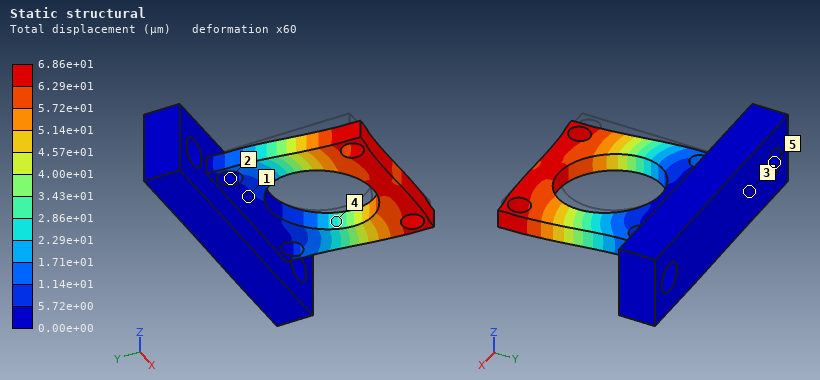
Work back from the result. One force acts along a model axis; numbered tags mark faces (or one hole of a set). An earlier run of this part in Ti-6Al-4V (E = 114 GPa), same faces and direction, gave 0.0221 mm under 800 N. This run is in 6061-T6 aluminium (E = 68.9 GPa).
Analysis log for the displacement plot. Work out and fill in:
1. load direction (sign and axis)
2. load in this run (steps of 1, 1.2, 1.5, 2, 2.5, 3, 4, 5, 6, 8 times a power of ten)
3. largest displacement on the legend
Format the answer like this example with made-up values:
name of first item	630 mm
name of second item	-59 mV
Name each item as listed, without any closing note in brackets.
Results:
load direction	+X
load in this run	1.5 kN
largest displacement on the legend	6.86e+01 µm
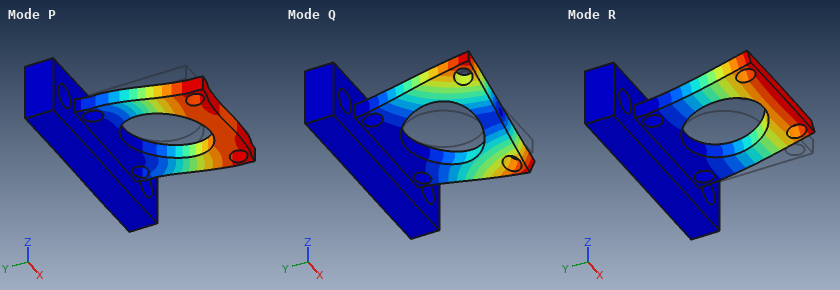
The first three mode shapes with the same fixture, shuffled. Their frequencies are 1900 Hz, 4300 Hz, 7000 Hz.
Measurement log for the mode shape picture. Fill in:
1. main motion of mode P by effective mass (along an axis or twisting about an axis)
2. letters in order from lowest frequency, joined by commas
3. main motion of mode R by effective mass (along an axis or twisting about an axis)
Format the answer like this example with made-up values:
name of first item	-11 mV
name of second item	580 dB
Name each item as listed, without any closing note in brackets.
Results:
main motion of mode P by effective mass	along X
letters in order from lowest frequency, joined by commas	R, Q, P
main motion of mode R by effective mass	along Z
